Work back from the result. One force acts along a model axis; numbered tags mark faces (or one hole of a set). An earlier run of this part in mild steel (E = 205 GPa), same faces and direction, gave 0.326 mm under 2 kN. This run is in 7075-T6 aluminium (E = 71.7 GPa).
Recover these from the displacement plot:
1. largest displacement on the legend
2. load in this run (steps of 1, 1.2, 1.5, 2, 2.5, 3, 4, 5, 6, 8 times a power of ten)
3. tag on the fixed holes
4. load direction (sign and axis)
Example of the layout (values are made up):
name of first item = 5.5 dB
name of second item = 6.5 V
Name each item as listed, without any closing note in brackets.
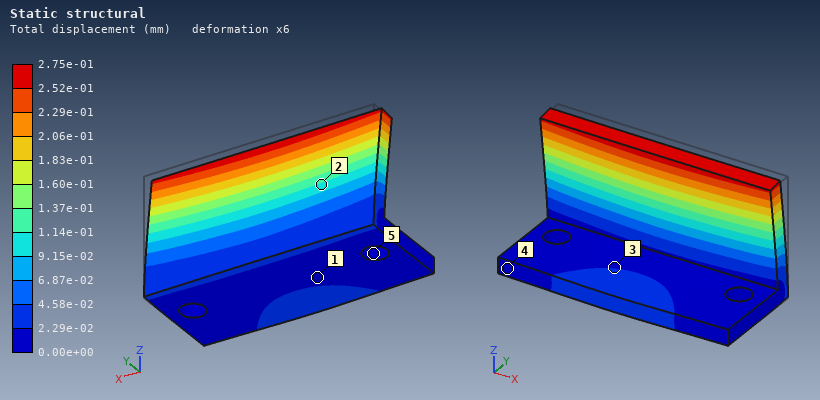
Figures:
largest displacement on the legend = 2.75e-01 mm
load in this run = 600 N
tag on the fixed holes = 5
load direction = -Y
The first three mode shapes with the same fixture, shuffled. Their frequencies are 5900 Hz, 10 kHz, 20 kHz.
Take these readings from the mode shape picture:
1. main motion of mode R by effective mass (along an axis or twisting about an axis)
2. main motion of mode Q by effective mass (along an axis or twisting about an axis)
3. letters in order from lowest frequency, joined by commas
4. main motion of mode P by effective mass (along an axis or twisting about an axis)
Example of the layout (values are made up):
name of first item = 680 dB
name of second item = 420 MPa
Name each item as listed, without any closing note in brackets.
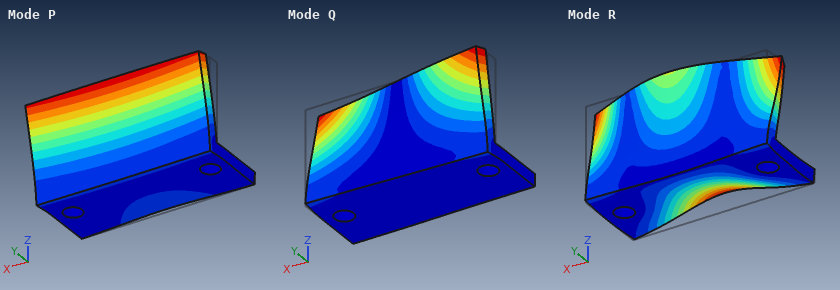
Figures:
main motion of mode R by effective mass = along Z
main motion of mode Q by effective mass = twisting about Z
letters in order from lowest frequency, joined by commas = P, Q, R
main motion of mode P by effective mass = along Y
